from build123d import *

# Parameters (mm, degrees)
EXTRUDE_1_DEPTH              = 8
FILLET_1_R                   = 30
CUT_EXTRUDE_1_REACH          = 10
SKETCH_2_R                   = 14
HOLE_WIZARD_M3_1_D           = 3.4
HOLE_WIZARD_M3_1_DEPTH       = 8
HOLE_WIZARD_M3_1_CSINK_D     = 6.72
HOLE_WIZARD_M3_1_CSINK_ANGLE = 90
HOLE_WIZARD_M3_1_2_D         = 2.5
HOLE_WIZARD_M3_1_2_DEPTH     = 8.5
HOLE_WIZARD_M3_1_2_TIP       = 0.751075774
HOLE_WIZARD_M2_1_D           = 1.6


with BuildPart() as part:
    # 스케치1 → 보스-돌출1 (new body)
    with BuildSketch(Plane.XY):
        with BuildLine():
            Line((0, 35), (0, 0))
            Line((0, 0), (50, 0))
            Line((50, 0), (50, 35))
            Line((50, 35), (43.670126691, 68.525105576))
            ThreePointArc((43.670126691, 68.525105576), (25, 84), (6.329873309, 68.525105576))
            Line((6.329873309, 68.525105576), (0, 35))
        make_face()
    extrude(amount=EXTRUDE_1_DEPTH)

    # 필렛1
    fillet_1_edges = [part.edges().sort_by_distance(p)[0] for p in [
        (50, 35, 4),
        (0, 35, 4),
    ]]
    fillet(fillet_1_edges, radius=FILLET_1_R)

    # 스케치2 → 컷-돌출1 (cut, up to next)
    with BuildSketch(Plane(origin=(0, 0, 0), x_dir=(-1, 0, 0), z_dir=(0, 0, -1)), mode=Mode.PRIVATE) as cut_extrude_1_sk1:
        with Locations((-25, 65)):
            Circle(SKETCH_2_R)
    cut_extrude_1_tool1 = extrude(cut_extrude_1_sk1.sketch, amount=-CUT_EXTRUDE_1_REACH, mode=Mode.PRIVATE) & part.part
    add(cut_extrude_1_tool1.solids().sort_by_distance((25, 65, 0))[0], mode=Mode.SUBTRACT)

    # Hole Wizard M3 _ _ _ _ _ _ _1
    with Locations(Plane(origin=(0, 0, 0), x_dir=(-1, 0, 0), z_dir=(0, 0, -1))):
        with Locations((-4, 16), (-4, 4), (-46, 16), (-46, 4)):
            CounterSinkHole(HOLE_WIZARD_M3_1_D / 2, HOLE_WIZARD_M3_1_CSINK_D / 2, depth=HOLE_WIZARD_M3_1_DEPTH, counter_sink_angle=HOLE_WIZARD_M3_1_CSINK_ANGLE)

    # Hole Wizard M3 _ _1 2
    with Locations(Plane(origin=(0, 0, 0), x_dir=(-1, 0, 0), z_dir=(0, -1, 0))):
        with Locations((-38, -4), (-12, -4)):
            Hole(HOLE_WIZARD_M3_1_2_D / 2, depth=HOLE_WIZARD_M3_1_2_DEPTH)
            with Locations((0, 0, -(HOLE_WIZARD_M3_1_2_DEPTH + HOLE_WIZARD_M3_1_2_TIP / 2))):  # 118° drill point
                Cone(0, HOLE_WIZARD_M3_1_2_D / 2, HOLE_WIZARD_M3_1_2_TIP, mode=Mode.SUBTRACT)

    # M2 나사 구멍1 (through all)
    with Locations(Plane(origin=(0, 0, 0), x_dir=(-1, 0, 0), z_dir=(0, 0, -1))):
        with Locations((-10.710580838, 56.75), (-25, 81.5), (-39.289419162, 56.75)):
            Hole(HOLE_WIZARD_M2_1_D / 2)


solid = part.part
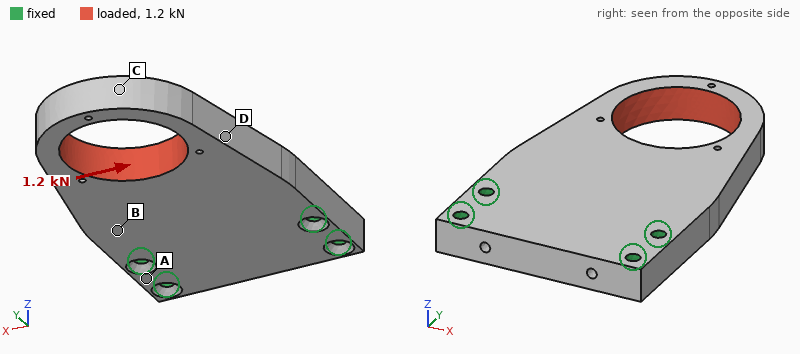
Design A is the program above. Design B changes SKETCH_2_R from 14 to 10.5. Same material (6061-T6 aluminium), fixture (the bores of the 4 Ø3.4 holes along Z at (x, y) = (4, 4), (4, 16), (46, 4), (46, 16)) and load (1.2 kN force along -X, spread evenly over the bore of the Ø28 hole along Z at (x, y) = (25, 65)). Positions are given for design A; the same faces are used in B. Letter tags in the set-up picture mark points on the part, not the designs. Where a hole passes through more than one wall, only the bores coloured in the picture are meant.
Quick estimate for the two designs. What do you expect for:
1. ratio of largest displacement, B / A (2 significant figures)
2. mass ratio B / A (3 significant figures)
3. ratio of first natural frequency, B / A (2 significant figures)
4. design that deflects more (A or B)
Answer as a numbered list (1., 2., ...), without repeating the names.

1. 0.51
2. 1.09
3. 0.87
4. A
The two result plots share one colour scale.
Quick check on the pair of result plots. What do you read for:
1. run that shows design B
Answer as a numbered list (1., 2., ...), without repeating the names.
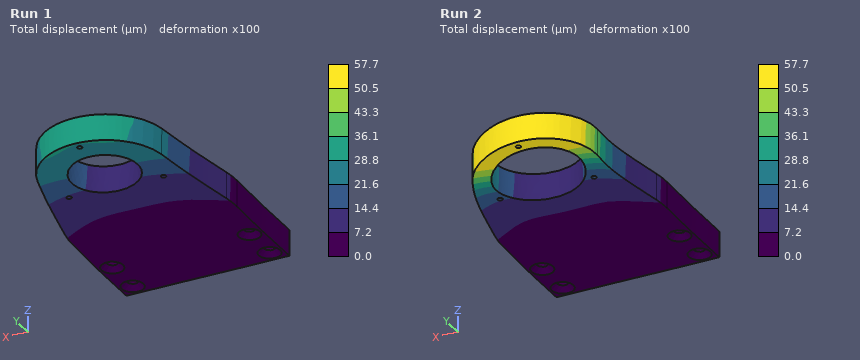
1. Run 1
